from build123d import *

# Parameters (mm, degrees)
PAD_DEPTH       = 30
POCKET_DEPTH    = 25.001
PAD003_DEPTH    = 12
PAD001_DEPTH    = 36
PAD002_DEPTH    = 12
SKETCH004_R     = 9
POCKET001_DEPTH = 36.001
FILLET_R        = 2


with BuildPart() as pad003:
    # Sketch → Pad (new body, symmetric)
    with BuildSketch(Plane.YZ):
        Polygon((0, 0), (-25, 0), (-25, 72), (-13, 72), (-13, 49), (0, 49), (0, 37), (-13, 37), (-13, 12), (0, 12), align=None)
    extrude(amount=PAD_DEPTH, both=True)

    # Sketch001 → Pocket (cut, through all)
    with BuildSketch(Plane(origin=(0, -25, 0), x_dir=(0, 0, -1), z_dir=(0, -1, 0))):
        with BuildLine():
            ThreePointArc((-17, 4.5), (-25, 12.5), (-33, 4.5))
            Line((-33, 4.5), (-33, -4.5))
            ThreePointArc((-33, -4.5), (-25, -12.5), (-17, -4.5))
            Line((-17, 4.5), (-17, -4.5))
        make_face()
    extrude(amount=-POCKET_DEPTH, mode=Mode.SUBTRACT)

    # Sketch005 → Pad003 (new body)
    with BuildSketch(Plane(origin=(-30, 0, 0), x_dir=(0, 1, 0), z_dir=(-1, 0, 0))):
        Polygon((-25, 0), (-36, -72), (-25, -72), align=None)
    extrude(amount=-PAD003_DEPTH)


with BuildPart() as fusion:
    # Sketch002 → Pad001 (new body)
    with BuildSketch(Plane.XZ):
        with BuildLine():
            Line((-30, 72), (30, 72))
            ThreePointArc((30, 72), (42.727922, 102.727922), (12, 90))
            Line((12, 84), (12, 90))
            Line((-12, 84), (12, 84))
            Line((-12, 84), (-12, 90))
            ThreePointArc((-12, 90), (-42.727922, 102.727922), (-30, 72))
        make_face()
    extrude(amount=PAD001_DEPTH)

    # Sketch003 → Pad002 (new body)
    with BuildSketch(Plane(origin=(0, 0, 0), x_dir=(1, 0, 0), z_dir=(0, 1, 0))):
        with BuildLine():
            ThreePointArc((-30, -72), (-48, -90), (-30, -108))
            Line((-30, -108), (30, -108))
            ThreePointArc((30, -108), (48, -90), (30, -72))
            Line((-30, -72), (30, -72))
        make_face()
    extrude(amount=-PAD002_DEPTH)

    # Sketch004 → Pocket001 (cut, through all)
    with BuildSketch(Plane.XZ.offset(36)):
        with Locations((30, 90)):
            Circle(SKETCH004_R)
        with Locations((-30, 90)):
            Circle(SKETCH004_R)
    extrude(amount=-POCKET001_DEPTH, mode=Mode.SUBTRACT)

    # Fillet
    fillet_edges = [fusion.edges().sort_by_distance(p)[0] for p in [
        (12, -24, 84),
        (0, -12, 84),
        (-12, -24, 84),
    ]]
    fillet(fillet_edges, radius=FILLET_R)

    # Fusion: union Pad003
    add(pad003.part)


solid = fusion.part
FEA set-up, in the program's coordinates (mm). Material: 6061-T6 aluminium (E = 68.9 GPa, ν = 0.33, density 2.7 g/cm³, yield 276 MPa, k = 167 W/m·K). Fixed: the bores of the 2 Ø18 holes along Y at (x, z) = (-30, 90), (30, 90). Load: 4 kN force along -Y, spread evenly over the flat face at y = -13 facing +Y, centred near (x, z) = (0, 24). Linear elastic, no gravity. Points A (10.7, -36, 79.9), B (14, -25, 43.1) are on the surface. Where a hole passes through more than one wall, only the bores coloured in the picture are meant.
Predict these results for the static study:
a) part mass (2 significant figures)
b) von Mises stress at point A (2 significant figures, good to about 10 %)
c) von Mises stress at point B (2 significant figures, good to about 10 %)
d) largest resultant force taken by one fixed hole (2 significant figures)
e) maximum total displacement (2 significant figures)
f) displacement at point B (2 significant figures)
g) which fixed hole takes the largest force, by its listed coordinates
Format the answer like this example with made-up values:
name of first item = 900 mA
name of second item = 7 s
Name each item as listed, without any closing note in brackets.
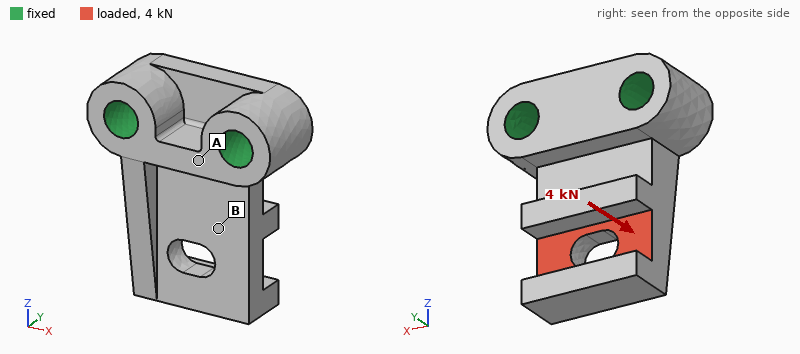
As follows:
part mass = 410 g
von Mises stress at point A = 14 MPa
von Mises stress at point B = 29 MPa
largest resultant force taken by one fixed hole = 2.2 kN
maximum total displacement = 0.35 mm
displacement at point B = 0.100 mm
which fixed hole takes the largest force, by its listed coordinates = (-30, 90)
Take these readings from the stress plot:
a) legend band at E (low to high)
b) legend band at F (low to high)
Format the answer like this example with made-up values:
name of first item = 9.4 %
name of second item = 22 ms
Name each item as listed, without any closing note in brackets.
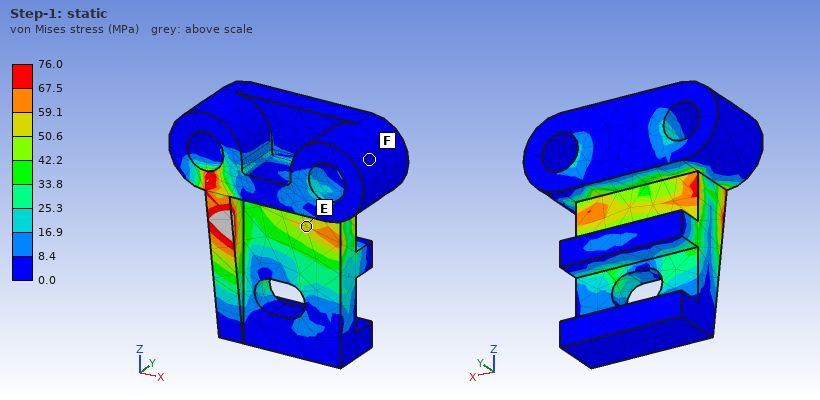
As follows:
legend band at E = 50.6 to 59.1 MPa
legend band at F = 0.0 to 8.4 MPa
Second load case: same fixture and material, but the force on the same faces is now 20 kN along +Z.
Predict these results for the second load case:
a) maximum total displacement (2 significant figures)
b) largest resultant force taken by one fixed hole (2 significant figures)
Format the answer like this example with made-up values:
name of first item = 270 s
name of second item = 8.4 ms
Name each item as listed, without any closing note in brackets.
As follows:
maximum total displacement = 0.41 mm
largest resultant force taken by one fixed hole = 11 kN
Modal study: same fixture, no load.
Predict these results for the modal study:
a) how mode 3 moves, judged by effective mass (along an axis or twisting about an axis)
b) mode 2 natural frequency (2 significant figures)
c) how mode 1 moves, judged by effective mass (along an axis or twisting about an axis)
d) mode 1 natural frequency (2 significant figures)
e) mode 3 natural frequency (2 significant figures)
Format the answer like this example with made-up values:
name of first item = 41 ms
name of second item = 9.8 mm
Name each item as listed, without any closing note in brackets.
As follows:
how mode 3 moves, judged by effective mass = along X
mode 2 natural frequency = 4100 Hz
how mode 1 moves, judged by effective mass = along Y
mode 1 natural frequency = 1700 Hz
mode 3 natural frequency = 5000 Hz
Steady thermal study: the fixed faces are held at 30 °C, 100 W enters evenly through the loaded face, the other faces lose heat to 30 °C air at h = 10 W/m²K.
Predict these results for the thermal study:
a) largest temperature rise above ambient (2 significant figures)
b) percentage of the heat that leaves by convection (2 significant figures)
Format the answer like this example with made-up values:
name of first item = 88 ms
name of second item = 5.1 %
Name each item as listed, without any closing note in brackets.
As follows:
largest temperature rise above ambient = 47 K
percentage of the heat that leaves by convection = 4.6 %
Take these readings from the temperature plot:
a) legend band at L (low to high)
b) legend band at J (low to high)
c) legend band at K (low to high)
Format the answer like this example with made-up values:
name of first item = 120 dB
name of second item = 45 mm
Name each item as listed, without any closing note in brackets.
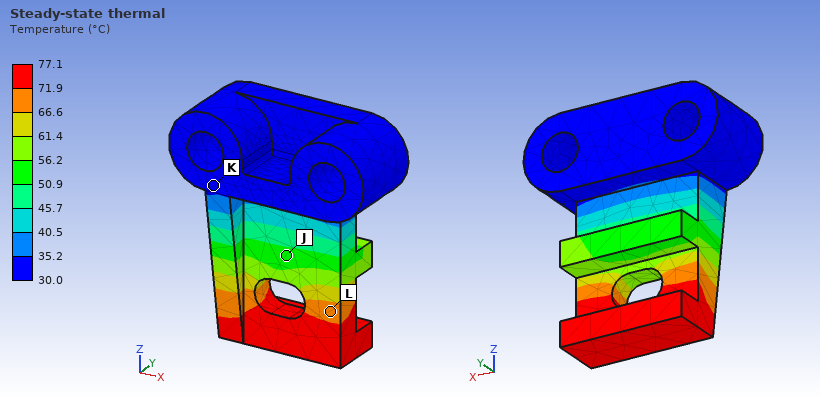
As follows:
legend band at L = 66.6 to 71.9 °C
legend band at J = 50.9 to 56.2 °C
legend band at K = 30.0 to 35.2 °C
